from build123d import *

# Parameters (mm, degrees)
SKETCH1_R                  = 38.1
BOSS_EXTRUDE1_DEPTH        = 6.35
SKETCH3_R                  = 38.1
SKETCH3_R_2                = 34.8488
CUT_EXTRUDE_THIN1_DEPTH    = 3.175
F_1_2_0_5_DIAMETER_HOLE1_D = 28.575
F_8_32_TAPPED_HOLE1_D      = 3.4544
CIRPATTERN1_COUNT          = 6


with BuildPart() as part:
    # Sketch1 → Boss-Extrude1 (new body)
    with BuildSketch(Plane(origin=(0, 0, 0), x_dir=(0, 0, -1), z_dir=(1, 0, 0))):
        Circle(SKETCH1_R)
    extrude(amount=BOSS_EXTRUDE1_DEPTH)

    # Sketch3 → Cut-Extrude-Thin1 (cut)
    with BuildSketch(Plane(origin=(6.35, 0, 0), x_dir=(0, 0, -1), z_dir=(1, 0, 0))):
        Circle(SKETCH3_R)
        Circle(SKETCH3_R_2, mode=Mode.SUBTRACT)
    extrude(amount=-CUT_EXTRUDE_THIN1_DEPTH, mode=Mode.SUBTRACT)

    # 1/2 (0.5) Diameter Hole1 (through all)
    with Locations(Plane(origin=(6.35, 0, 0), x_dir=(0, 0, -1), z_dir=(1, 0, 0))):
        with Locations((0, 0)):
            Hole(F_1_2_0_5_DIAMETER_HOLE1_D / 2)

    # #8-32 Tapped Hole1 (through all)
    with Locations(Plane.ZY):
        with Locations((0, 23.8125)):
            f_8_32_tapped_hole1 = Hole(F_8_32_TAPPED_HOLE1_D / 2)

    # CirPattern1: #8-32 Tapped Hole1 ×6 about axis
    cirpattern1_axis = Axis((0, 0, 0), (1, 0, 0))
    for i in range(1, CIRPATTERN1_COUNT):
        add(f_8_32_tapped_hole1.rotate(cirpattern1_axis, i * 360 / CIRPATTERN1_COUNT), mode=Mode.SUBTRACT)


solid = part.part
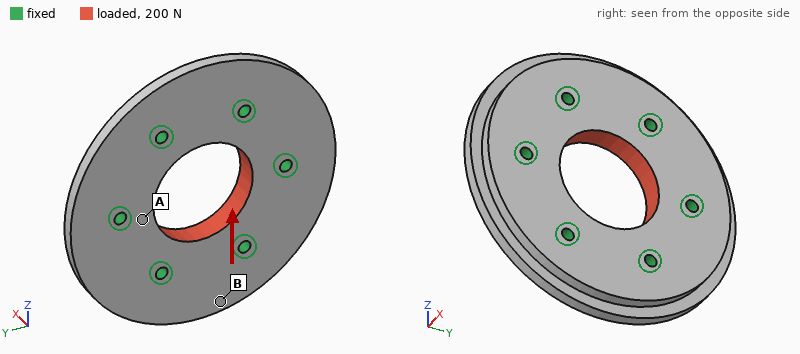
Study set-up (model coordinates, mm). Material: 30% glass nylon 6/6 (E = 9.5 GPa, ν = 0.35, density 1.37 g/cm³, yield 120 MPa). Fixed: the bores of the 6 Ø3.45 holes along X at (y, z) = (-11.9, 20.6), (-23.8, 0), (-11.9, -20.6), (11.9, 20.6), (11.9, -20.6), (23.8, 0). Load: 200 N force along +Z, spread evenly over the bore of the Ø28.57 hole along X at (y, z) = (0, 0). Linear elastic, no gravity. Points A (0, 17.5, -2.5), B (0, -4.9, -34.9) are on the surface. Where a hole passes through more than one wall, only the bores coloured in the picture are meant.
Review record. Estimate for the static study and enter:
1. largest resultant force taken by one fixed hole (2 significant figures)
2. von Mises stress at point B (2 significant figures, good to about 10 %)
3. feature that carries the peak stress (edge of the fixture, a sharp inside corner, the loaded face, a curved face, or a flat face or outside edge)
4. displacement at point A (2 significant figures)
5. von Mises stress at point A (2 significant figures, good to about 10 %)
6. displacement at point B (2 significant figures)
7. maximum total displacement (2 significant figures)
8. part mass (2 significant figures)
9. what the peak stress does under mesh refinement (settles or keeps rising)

39 N
0.099 MPa
edge of the fixture
0.38 µm
0.31 MPa
0.28 µm
0.69 µm
30 g
keeps rising
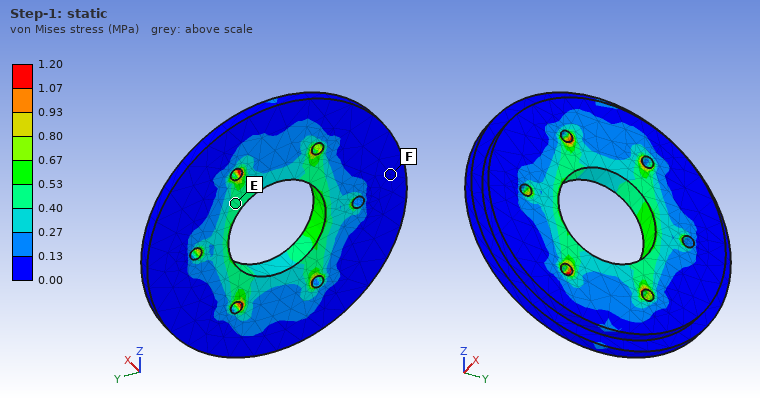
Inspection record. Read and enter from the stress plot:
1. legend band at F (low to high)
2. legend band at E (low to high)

0.00 to 0.13 MPa
0.40 to 0.53 MPa
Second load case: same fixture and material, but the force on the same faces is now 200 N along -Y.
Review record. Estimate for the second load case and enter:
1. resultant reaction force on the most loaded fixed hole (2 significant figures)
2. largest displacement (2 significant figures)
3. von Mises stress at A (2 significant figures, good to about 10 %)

43 N
0.68 µm
0.47 MPa
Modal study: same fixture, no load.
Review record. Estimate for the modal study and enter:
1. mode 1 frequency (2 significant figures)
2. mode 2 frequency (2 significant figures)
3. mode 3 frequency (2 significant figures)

9400 Hz
9600 Hz
9600 Hz
